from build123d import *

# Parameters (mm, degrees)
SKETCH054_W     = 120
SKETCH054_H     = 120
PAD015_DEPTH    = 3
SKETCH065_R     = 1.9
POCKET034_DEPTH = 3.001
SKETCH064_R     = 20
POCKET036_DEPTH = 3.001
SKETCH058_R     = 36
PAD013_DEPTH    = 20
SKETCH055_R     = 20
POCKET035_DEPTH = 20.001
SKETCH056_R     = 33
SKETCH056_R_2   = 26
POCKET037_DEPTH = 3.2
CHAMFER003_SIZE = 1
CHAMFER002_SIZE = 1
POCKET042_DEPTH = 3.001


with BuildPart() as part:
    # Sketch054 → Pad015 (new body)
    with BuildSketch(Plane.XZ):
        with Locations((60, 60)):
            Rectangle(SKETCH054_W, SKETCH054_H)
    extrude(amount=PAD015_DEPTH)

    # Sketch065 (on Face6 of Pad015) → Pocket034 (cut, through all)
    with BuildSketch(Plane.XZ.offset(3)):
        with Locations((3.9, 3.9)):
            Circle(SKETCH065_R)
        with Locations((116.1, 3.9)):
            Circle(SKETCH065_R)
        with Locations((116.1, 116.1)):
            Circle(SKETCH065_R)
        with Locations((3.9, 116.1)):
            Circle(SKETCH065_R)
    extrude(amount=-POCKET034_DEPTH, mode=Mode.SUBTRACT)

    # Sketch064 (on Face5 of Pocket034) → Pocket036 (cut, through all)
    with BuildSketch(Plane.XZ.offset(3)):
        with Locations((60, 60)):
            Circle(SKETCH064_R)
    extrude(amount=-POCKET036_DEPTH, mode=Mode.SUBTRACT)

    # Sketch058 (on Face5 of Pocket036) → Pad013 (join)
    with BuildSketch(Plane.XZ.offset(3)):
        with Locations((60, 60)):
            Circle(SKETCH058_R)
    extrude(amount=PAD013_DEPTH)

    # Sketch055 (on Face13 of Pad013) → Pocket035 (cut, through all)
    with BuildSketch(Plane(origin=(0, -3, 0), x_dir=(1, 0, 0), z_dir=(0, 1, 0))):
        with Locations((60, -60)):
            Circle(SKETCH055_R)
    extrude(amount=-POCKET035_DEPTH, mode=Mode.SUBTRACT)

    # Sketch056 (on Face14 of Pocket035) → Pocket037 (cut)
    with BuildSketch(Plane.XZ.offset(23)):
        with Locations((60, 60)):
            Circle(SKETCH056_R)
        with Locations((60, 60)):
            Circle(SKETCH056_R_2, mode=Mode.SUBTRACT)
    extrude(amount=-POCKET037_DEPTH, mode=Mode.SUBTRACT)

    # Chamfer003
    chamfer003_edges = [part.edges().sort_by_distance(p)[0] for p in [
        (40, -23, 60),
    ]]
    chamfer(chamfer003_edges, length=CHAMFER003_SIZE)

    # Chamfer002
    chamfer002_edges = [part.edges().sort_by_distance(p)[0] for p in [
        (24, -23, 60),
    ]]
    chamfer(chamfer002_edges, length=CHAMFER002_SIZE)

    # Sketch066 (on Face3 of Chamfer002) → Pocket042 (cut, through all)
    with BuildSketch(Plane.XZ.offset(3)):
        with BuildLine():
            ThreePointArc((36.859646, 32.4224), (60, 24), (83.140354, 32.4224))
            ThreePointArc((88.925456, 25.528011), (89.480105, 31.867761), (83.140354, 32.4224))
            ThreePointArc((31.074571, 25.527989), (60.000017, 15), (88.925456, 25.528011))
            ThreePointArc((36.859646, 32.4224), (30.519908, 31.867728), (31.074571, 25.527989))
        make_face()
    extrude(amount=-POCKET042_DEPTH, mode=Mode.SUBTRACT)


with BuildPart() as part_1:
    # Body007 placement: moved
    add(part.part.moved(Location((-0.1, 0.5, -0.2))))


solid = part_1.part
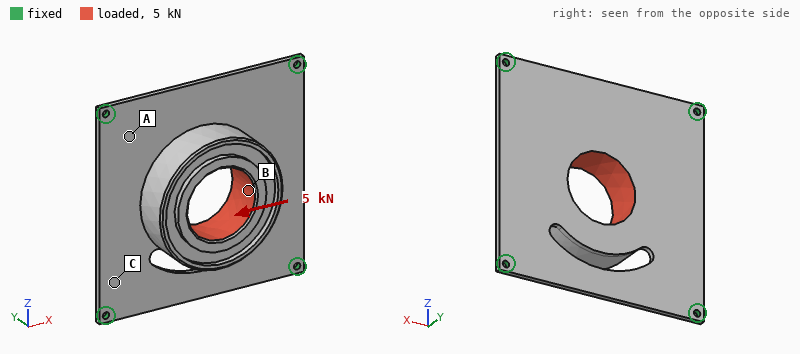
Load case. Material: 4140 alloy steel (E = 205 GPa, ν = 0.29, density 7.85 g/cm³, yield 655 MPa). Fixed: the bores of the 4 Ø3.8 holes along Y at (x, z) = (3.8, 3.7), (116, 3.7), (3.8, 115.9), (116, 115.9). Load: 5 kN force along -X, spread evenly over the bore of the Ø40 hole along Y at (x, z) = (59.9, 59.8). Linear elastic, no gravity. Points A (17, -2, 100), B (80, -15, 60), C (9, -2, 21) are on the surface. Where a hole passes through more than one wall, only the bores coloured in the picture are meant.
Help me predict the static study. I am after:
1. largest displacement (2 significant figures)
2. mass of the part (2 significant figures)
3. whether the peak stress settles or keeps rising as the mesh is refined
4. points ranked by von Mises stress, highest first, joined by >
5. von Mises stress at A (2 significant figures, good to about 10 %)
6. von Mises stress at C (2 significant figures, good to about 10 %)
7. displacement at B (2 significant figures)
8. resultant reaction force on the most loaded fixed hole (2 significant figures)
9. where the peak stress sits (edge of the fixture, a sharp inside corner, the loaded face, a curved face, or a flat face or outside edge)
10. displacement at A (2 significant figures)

0.15 mm
700 g
keeps rising
A > C > B
52 MPa
34 MPa
0.074 mm
2.0 kN
edge of the fixture
0.053 mm
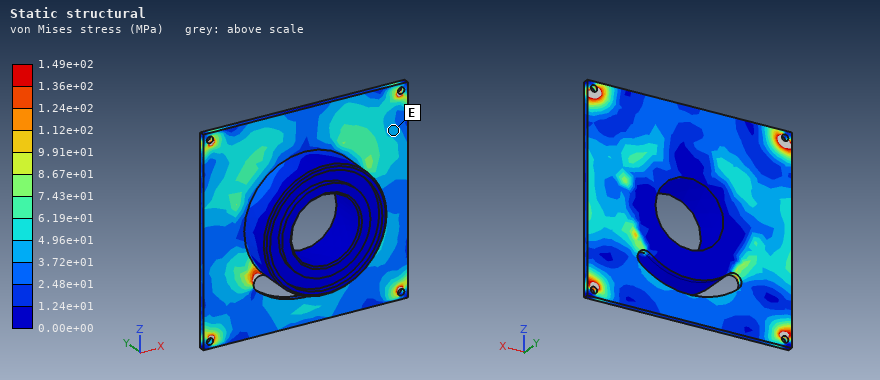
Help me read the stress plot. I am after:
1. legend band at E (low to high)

3.72e+01 to 4.96e+01 MPa
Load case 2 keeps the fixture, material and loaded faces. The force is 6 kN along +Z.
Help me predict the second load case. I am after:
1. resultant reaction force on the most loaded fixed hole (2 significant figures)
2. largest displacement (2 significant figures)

1.8 kN
0.23 mm
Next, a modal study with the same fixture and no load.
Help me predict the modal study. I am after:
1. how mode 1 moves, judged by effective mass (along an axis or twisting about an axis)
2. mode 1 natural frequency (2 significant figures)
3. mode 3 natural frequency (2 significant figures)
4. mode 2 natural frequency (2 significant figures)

along Y
530 Hz
1000 Hz
990 Hz
